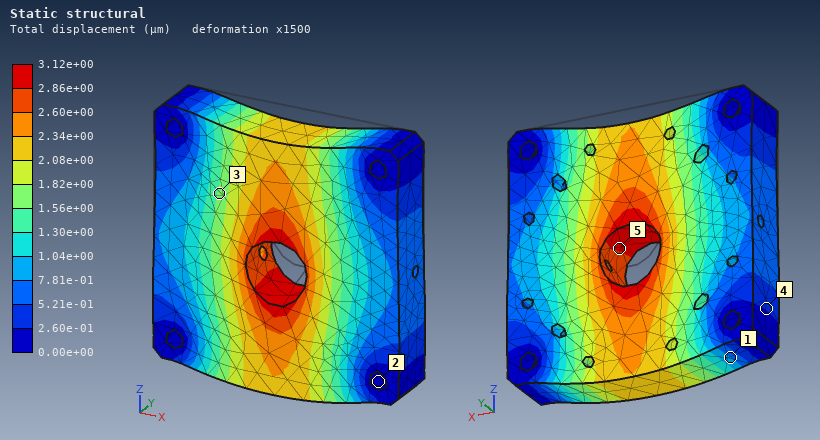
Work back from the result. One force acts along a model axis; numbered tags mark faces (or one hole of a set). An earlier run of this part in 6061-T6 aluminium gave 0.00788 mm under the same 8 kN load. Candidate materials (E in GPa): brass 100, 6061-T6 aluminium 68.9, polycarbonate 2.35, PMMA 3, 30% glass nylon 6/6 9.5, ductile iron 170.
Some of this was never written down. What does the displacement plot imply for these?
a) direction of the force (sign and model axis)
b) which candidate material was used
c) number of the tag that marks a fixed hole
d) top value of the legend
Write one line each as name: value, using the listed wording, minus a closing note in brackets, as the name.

direction of the force: -Z
which candidate material was used: ductile iron
number of the tag that marks a fixed hole: 2
top value of the legend: 3.12e+00 µm
